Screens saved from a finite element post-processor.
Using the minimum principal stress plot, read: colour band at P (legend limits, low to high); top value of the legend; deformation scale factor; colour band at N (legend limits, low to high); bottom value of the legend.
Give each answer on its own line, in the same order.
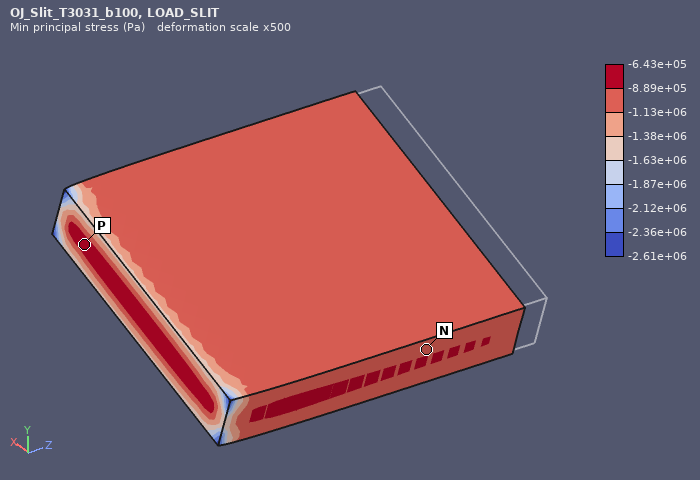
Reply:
-8.89e+05 to -6.43e+05 Pa
-6.43e+05 Pa
500
-1.13e+06 to -8.89e+05 Pa
-2.61e+06 Pa
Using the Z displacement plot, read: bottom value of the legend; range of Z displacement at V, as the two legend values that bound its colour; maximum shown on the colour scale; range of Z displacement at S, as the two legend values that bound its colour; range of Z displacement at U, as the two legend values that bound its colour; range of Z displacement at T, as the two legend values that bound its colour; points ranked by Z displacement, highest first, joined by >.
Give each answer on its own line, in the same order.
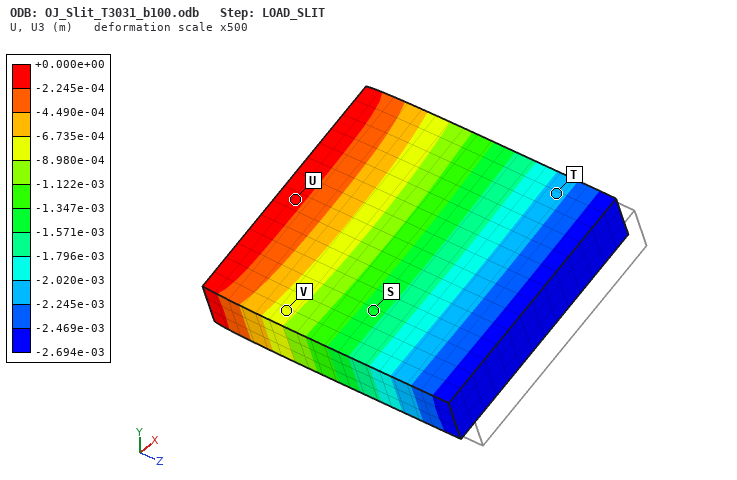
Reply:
-2.694e-03 m
-8.980e-04 to -6.735e-04 m
+0.000e+00 m
-1.571e-03 to -1.347e-03 m
-2.245e-04 to +0.000e+00 m
-2.245e-03 to -2.020e-03 m
U > V > S > T
